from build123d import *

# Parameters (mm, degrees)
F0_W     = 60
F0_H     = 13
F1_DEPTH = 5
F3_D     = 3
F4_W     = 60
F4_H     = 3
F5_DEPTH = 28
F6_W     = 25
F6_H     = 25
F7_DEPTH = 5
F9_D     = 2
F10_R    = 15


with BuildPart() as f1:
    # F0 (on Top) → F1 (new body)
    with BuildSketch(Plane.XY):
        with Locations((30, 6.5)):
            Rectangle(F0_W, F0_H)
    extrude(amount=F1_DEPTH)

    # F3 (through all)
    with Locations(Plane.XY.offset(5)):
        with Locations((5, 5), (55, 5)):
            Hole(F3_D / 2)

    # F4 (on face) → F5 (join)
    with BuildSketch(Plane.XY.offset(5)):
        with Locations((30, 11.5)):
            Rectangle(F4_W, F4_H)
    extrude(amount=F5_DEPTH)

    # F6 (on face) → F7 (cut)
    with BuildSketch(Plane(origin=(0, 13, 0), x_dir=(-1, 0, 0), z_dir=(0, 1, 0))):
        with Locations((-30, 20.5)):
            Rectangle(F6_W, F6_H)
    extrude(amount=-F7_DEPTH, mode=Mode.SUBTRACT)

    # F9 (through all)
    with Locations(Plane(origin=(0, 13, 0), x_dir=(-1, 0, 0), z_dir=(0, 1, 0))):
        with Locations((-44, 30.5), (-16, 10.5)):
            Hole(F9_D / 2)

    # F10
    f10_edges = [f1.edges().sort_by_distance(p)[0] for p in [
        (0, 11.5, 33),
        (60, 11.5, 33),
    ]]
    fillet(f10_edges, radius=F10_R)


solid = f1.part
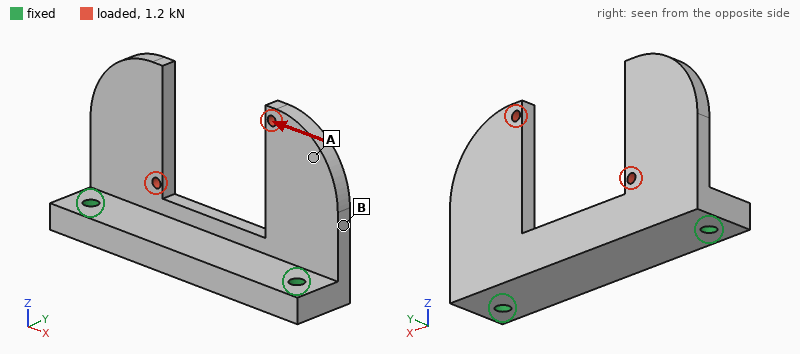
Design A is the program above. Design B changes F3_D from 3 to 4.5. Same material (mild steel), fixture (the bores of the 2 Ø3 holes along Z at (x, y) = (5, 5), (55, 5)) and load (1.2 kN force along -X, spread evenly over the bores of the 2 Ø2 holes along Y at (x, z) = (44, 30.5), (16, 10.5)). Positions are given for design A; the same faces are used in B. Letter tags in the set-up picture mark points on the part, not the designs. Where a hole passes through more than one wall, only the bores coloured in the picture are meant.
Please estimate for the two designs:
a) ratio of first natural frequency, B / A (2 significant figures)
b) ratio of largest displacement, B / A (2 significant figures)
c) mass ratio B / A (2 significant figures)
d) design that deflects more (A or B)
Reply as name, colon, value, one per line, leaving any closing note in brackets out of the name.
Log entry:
ratio of first natural frequency, B / A: 1.0
ratio of largest displacement, B / A: 0.91
mass ratio B / A: 0.99
design that deflects more: A
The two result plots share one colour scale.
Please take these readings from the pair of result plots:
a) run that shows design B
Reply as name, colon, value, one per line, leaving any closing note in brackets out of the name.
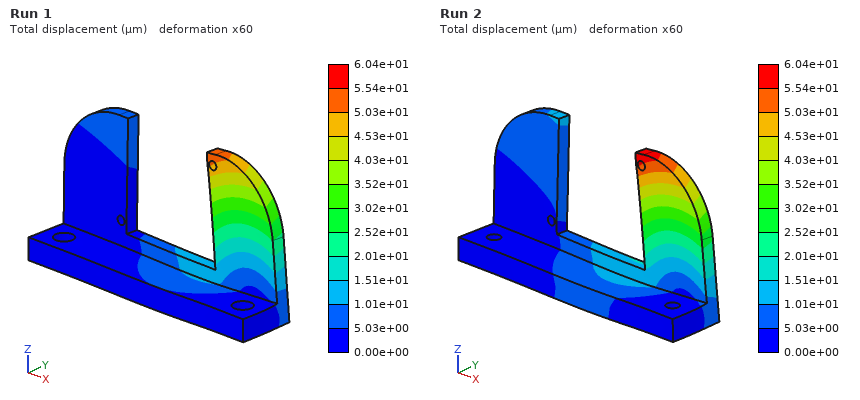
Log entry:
run that shows design B: Run 1
